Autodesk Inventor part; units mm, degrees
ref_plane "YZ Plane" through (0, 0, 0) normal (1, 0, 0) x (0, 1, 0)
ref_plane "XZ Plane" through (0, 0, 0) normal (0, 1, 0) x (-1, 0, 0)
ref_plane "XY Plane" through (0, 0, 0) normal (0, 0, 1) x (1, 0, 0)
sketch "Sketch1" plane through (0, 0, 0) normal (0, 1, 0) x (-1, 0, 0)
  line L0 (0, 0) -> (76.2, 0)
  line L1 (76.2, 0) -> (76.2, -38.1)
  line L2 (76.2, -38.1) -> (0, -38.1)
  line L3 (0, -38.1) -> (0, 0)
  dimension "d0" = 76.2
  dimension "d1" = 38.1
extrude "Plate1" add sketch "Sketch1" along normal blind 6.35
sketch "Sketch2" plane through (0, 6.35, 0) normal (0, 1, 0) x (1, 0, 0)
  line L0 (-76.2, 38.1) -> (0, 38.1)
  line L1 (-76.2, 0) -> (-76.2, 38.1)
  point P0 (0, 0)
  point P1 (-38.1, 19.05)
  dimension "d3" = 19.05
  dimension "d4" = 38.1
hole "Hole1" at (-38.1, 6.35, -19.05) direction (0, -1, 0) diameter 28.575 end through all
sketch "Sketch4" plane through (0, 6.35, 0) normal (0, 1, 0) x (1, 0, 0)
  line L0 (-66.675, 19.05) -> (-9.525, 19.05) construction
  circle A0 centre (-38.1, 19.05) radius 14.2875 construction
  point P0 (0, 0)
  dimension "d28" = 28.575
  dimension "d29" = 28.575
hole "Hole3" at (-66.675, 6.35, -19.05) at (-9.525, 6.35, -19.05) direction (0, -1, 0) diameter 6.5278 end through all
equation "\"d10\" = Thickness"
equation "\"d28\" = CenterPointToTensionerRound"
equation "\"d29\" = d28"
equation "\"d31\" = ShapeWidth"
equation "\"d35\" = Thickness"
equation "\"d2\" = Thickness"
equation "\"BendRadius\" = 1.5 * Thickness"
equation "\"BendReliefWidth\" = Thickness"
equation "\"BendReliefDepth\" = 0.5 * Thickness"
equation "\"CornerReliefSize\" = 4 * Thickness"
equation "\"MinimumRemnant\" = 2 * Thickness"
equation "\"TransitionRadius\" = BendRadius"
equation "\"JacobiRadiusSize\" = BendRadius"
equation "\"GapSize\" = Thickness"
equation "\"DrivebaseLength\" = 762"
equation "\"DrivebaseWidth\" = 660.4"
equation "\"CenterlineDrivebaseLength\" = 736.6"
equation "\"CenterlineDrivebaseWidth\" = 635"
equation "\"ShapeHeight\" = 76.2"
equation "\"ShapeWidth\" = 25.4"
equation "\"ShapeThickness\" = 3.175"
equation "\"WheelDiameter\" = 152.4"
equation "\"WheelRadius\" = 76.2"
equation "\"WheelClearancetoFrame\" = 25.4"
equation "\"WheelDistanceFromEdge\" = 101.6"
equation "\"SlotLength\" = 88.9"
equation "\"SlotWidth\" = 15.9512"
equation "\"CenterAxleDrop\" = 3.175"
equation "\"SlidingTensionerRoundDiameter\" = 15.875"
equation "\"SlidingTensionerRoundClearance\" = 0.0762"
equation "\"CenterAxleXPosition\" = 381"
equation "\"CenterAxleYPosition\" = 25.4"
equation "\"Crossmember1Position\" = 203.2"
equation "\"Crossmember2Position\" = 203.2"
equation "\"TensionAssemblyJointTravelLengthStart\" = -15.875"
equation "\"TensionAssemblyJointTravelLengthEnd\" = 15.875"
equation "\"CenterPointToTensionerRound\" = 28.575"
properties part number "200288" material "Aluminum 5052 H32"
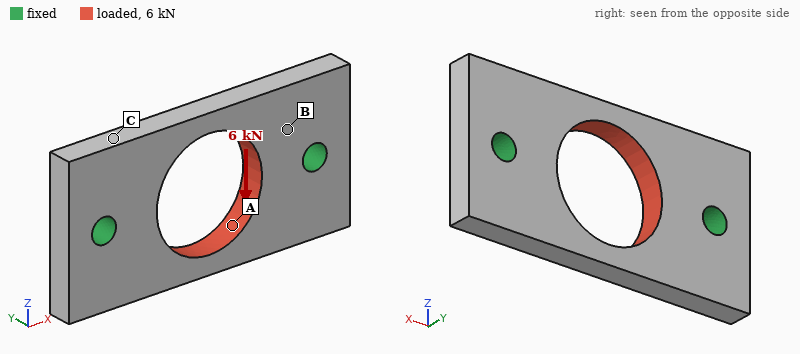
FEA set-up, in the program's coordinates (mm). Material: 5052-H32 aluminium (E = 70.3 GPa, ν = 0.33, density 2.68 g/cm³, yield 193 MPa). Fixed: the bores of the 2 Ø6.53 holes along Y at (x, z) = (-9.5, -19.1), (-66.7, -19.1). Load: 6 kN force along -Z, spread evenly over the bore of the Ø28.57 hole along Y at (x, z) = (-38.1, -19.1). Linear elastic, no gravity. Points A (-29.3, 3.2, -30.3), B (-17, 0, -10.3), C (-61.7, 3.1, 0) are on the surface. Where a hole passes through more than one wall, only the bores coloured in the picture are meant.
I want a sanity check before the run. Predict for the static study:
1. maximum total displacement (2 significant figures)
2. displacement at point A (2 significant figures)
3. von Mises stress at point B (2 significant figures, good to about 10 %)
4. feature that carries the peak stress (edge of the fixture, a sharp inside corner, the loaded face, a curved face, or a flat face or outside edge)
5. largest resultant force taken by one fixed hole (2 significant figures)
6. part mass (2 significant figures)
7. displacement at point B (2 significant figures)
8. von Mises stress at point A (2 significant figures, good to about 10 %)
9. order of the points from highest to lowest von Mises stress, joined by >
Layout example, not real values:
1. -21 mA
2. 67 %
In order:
1. 28 µm
2. 20 µm
3. 25 MPa
4. edge of the fixture
5. 3.0 kN
6. 37 g
7. 7.4 µm
8. 48 MPa
9. A > B > C
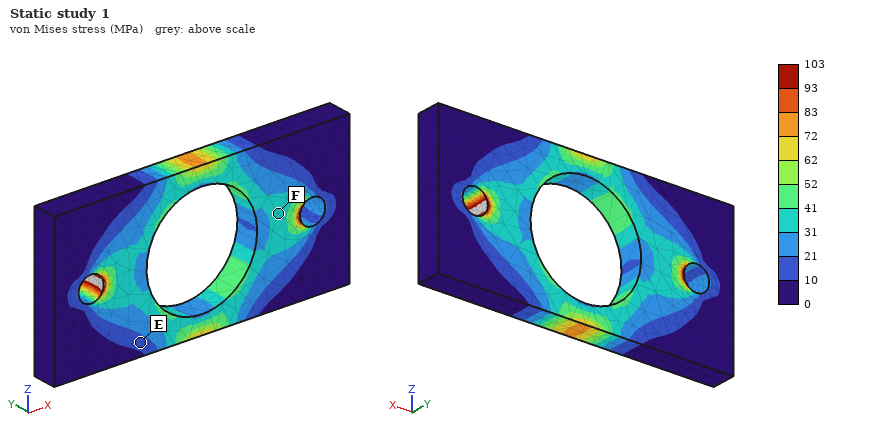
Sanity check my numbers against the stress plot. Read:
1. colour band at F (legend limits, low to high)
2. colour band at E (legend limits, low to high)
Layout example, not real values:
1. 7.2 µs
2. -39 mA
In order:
1. 31 to 41 MPa
2. 10 to 21 MPa
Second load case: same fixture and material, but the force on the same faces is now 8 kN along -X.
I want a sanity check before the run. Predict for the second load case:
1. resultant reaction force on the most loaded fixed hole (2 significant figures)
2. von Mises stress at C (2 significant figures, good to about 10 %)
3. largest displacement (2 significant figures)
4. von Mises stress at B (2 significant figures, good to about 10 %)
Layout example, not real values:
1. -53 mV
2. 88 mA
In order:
1. 4.0 kN
2. 7.6 MPa
3. 14 µm
4. 24 MPa
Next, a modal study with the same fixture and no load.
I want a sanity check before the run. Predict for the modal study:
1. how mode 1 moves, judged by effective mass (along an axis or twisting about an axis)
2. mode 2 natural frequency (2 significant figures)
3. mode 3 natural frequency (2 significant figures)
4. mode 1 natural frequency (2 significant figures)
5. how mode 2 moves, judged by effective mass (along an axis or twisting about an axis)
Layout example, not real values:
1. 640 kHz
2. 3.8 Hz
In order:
1. twisting about X
2. 9500 Hz
3. 14 kHz
4. 8600 Hz
5. along Y
